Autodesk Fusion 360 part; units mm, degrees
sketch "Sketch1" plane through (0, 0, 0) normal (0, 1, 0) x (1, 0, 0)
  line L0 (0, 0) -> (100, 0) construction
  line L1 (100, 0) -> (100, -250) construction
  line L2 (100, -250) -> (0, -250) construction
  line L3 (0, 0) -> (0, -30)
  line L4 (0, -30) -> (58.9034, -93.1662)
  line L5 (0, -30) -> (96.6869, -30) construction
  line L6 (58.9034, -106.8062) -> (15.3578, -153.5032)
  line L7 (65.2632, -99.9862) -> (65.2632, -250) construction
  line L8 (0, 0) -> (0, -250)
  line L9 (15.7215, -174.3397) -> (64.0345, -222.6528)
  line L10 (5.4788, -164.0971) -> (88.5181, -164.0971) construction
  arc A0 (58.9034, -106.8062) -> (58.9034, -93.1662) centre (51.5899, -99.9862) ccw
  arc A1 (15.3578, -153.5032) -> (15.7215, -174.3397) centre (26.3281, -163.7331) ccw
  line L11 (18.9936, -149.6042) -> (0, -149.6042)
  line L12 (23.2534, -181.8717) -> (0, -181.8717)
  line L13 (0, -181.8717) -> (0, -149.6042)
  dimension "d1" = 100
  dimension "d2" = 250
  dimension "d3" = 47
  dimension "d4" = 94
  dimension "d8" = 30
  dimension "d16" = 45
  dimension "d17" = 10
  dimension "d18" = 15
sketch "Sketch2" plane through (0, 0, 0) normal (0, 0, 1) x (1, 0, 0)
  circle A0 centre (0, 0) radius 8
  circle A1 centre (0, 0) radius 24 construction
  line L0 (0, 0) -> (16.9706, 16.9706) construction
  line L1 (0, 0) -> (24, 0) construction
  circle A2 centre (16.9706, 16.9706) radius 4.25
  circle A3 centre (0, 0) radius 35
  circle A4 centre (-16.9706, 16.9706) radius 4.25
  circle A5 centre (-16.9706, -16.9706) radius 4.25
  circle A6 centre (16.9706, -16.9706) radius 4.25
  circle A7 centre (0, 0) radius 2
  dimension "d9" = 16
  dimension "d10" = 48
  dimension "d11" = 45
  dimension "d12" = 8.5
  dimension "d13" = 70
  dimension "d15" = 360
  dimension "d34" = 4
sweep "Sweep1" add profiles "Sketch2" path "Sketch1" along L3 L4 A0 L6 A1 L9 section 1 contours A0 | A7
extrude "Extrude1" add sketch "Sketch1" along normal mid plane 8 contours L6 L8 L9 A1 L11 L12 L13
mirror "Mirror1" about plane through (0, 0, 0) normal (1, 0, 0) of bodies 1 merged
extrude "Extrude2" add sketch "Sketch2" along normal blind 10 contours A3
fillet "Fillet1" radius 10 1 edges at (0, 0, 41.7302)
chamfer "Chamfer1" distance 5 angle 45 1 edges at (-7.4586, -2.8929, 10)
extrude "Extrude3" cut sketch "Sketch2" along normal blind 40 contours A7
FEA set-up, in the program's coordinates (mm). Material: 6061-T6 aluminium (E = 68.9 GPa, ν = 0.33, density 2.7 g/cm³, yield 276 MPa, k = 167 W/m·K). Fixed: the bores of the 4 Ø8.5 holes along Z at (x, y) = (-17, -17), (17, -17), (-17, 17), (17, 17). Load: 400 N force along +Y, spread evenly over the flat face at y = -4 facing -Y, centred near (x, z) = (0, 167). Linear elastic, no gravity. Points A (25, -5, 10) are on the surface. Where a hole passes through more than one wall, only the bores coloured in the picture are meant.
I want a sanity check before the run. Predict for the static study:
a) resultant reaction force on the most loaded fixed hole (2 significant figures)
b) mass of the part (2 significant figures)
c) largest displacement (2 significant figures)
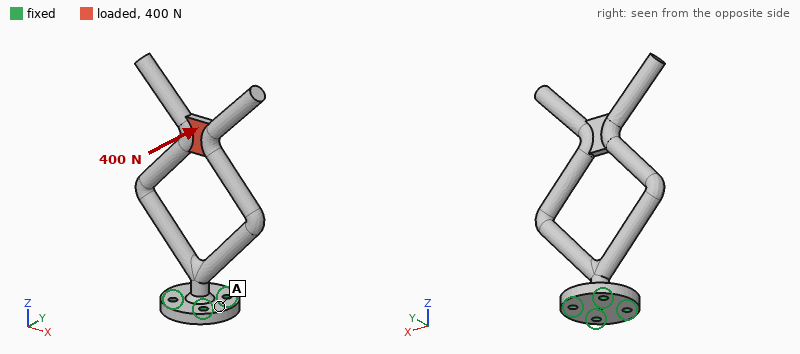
1.1 kN
390 g
3.1 mm
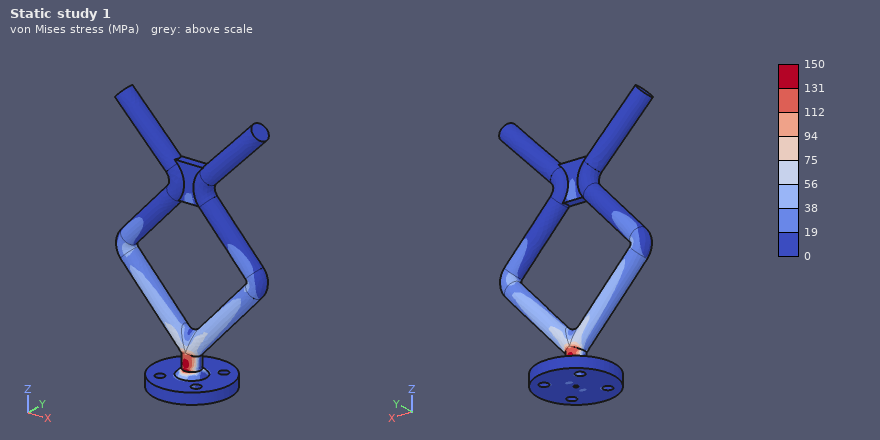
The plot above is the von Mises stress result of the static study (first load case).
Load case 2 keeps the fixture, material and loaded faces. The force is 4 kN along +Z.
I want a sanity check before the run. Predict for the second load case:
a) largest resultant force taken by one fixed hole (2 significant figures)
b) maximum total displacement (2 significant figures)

1.3 kN
1.3 mm
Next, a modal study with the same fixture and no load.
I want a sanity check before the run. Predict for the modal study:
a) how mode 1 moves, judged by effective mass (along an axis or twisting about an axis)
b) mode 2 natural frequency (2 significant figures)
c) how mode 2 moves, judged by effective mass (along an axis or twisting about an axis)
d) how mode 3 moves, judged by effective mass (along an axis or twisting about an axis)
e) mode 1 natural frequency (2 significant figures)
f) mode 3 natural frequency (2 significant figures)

along Y
200 Hz
along X
twisting about Z
160 Hz
470 Hz
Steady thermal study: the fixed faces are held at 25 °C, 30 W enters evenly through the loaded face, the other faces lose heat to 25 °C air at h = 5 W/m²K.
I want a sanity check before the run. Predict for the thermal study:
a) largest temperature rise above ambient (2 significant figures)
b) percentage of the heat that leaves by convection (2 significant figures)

82 K
25 %
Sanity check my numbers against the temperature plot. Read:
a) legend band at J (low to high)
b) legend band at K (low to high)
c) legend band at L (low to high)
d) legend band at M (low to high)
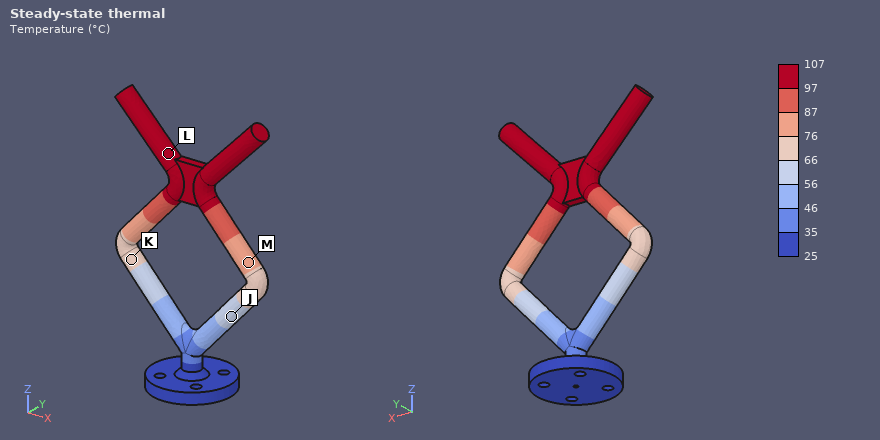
56 to 66 °C
66 to 76 °C
97 to 107 °C
76 to 87 °C
